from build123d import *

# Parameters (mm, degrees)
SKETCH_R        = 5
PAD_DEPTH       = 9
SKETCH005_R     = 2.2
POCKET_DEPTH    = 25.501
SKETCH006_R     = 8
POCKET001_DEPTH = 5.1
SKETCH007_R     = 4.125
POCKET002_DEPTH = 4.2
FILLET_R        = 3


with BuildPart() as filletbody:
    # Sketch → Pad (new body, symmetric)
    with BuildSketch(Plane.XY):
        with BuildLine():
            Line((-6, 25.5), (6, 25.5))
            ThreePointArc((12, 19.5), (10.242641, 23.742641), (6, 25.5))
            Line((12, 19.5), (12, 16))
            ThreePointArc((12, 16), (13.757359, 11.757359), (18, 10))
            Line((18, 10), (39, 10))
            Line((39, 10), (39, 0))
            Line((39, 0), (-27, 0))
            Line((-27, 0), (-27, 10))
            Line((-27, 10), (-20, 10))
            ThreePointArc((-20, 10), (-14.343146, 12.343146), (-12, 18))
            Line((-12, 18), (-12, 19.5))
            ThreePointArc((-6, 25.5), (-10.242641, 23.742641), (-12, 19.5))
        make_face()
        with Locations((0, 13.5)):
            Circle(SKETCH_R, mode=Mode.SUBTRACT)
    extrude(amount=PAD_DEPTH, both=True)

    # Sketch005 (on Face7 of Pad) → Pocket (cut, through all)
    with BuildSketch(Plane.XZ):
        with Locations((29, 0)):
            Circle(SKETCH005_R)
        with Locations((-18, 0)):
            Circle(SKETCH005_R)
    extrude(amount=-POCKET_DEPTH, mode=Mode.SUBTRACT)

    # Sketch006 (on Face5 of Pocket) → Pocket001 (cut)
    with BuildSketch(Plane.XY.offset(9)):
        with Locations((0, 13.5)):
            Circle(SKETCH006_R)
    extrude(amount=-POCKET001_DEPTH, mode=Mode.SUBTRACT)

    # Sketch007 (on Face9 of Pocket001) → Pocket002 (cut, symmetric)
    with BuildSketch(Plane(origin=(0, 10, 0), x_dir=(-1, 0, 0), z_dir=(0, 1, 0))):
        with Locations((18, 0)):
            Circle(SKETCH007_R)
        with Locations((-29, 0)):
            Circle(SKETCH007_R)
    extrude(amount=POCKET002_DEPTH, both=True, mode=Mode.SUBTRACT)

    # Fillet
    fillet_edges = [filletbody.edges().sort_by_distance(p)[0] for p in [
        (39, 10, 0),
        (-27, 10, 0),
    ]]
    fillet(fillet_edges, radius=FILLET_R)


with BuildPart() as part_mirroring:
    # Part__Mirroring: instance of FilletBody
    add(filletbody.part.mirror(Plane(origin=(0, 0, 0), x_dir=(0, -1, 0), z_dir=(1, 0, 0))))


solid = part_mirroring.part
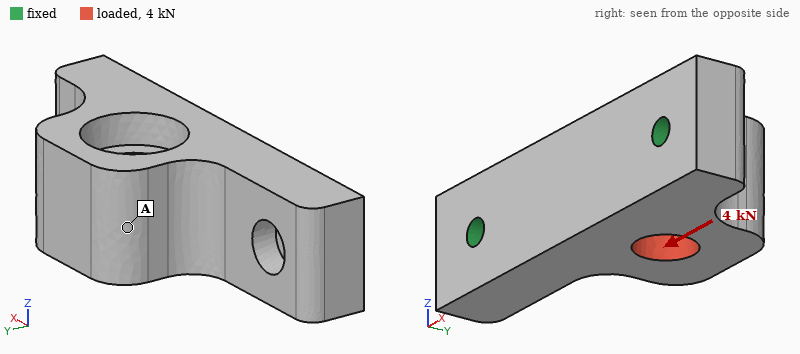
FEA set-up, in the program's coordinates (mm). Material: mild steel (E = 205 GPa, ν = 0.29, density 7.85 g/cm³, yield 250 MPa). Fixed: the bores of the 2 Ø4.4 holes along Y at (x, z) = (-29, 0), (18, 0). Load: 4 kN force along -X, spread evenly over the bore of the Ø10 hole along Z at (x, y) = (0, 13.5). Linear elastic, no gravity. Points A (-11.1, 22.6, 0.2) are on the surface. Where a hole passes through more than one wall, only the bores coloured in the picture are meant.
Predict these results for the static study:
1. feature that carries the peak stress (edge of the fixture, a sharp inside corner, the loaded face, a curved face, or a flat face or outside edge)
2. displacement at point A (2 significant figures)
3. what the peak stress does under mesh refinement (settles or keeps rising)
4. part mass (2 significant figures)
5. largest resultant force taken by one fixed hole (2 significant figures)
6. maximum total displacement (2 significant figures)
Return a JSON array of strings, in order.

["edge of the fixture", "4.3 µm", "keeps rising", "120 g", "2.2 kN", "4.7 µm"]
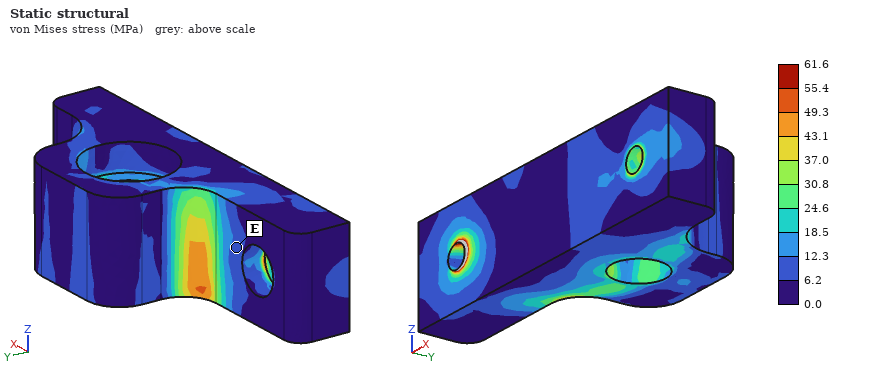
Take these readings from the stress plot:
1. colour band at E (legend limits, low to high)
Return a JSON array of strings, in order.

["6.2 to 12.3 MPa"]
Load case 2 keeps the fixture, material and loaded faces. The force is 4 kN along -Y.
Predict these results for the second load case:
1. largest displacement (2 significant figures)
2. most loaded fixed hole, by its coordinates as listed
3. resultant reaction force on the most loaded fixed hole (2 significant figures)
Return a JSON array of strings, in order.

["13 µm", "(18, 0)", "2.7 kN"]
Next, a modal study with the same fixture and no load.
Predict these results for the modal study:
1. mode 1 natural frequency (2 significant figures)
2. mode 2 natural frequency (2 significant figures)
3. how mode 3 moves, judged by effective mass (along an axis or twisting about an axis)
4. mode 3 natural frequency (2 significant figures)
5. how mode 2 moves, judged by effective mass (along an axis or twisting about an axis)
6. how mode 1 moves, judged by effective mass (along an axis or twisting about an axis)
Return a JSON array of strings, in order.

["7500 Hz", "13 kHz", "along Z", "18 kHz", "along Y", "along Z"]
